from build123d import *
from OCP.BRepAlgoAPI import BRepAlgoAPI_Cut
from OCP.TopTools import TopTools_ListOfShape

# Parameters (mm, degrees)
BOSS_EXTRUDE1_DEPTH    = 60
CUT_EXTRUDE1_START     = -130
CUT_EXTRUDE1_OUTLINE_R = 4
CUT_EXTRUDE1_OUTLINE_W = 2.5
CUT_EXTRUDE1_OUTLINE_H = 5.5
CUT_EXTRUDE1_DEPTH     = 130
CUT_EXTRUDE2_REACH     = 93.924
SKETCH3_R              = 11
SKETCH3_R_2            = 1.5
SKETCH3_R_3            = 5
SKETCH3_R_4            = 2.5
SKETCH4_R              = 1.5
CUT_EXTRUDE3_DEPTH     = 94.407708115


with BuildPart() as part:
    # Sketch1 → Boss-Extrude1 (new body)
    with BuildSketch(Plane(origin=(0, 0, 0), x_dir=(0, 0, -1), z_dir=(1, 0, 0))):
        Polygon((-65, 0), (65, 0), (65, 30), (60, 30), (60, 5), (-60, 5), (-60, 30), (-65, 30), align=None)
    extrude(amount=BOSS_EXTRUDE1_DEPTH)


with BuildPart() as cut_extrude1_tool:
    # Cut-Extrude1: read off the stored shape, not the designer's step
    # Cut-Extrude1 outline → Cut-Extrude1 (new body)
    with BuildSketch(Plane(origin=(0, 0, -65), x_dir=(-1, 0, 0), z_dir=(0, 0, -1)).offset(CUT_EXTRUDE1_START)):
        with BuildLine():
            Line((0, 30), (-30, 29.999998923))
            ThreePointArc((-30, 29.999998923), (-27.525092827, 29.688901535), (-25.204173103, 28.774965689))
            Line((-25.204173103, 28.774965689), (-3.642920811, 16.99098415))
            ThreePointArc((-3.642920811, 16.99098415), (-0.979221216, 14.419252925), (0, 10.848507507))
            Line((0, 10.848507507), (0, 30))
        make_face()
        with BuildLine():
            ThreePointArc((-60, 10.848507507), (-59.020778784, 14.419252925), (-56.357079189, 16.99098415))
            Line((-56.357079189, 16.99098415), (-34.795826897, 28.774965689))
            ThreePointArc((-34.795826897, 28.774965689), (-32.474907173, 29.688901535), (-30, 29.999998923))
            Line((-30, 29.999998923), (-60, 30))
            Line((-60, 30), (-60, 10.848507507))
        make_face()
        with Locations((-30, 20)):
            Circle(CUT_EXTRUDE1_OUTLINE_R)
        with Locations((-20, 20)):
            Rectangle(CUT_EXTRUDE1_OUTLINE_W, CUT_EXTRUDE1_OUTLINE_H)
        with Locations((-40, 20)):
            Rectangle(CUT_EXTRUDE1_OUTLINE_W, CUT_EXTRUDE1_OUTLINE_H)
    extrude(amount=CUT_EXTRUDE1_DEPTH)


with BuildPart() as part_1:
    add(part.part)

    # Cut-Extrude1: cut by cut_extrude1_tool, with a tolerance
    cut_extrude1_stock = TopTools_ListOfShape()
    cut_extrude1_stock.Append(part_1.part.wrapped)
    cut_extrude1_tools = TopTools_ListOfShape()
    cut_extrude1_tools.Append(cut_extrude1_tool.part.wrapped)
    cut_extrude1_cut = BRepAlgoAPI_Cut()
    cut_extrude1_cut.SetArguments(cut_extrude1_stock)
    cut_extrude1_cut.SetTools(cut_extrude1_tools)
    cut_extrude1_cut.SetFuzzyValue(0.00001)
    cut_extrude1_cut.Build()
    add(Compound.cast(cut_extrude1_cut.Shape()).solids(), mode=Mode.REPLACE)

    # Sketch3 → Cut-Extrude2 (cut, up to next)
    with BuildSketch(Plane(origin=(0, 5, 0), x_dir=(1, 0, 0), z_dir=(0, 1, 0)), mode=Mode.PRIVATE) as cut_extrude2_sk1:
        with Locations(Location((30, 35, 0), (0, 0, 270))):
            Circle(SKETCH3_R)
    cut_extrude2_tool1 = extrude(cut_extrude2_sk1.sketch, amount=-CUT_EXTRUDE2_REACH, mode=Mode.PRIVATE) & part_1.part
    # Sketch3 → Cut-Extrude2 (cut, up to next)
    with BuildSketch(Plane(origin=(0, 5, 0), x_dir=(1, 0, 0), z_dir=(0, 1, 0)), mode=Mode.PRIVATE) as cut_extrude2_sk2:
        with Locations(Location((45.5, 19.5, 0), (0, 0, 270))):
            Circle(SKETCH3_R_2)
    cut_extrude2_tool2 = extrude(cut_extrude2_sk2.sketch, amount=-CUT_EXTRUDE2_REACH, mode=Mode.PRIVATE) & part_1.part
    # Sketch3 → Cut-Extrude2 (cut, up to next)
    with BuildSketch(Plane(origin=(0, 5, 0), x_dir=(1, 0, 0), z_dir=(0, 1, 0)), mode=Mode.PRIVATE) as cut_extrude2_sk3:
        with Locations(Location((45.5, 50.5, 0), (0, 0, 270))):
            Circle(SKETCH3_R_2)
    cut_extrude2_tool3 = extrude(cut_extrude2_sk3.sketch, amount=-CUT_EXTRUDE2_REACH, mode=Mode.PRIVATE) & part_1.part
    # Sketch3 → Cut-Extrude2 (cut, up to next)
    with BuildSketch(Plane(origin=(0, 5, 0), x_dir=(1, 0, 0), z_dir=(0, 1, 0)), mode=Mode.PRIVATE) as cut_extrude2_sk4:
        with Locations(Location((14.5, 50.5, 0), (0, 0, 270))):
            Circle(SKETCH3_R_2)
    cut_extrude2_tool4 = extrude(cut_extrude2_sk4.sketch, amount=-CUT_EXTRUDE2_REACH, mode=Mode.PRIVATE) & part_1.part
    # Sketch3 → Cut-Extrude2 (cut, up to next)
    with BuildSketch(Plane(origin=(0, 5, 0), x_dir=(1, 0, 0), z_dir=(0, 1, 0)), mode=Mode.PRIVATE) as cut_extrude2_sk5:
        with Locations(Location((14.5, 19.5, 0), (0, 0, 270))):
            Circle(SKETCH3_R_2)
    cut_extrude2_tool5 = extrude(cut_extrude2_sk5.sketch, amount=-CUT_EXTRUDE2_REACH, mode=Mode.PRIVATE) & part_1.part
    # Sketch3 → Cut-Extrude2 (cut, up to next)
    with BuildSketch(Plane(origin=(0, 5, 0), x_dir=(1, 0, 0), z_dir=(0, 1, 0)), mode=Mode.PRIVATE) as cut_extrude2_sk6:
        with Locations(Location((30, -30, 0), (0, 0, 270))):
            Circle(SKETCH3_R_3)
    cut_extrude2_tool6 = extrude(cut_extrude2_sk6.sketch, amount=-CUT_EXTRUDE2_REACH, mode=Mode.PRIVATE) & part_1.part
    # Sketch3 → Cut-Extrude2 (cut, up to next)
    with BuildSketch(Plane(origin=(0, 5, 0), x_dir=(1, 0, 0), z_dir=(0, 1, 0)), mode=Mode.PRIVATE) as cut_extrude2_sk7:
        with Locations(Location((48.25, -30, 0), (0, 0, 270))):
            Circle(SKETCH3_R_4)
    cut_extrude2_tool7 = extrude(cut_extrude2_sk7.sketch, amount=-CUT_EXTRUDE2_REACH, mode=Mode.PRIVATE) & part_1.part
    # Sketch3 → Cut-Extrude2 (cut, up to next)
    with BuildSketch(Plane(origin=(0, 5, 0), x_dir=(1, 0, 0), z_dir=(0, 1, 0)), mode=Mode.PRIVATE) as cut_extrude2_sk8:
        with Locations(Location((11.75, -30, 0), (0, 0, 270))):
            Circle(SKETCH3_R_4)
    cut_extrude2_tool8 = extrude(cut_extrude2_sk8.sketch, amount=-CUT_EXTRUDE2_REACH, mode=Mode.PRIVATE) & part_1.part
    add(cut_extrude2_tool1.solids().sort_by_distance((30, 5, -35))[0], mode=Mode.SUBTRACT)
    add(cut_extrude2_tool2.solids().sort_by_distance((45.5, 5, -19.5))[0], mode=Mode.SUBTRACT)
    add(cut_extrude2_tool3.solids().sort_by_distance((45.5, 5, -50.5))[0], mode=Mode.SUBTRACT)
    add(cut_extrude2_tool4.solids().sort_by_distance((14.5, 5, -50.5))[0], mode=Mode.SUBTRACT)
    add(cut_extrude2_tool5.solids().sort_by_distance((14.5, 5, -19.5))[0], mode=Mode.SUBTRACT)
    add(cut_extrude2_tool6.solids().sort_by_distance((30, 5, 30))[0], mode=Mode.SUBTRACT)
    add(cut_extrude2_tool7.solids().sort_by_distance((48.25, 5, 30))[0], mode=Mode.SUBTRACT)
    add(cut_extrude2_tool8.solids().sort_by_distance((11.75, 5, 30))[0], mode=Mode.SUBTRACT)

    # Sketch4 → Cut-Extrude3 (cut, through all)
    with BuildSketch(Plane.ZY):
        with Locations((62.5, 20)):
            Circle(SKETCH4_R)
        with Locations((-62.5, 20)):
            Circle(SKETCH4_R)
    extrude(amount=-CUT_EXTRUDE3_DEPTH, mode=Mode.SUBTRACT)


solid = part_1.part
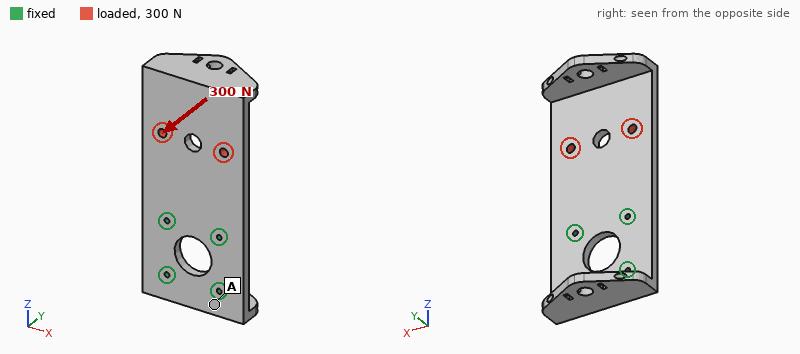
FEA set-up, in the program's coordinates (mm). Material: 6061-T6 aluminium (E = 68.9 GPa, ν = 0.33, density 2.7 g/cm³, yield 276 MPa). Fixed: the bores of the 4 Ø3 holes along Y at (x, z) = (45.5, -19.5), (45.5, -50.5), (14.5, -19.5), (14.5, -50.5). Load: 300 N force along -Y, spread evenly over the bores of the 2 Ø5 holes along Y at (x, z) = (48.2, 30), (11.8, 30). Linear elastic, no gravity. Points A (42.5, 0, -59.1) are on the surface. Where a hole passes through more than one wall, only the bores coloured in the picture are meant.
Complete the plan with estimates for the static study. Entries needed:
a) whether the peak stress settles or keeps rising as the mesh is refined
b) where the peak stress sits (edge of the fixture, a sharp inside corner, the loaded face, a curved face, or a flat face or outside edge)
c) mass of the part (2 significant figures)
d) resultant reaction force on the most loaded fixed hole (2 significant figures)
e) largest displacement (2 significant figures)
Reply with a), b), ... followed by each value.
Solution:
a) keeps rising
b) edge of the fixture
c) 120 g
d) 230 N
e) 0.69 mm
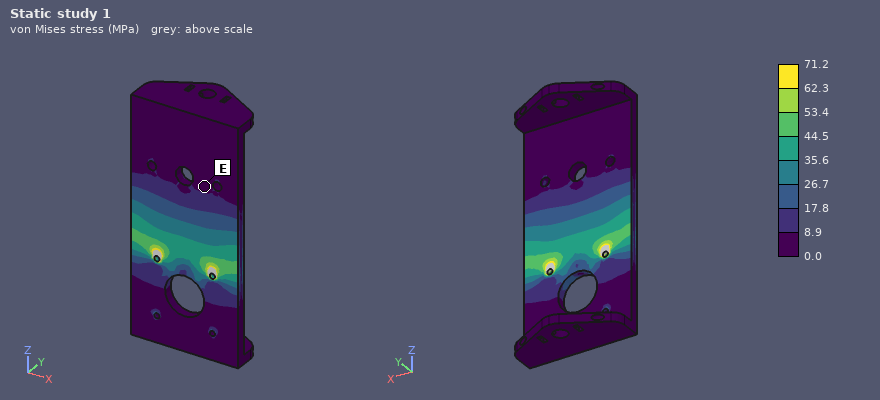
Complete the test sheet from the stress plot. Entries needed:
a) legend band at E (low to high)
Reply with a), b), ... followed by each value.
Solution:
a) 0.0 to 8.9 MPa
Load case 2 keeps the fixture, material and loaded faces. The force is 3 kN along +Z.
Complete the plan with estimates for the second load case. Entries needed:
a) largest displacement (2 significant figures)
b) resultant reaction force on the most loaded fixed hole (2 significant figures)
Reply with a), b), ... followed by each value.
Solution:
a) 11 µm
b) 1.3 kN
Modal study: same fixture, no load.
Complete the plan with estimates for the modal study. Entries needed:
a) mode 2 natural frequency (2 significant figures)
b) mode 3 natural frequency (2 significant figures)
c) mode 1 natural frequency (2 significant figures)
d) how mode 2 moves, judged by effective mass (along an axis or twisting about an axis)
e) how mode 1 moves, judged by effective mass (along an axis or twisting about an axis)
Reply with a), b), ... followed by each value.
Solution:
a) 1300 Hz
b) 2500 Hz
c) 420 Hz
d) twisting about Z
e) along Y
